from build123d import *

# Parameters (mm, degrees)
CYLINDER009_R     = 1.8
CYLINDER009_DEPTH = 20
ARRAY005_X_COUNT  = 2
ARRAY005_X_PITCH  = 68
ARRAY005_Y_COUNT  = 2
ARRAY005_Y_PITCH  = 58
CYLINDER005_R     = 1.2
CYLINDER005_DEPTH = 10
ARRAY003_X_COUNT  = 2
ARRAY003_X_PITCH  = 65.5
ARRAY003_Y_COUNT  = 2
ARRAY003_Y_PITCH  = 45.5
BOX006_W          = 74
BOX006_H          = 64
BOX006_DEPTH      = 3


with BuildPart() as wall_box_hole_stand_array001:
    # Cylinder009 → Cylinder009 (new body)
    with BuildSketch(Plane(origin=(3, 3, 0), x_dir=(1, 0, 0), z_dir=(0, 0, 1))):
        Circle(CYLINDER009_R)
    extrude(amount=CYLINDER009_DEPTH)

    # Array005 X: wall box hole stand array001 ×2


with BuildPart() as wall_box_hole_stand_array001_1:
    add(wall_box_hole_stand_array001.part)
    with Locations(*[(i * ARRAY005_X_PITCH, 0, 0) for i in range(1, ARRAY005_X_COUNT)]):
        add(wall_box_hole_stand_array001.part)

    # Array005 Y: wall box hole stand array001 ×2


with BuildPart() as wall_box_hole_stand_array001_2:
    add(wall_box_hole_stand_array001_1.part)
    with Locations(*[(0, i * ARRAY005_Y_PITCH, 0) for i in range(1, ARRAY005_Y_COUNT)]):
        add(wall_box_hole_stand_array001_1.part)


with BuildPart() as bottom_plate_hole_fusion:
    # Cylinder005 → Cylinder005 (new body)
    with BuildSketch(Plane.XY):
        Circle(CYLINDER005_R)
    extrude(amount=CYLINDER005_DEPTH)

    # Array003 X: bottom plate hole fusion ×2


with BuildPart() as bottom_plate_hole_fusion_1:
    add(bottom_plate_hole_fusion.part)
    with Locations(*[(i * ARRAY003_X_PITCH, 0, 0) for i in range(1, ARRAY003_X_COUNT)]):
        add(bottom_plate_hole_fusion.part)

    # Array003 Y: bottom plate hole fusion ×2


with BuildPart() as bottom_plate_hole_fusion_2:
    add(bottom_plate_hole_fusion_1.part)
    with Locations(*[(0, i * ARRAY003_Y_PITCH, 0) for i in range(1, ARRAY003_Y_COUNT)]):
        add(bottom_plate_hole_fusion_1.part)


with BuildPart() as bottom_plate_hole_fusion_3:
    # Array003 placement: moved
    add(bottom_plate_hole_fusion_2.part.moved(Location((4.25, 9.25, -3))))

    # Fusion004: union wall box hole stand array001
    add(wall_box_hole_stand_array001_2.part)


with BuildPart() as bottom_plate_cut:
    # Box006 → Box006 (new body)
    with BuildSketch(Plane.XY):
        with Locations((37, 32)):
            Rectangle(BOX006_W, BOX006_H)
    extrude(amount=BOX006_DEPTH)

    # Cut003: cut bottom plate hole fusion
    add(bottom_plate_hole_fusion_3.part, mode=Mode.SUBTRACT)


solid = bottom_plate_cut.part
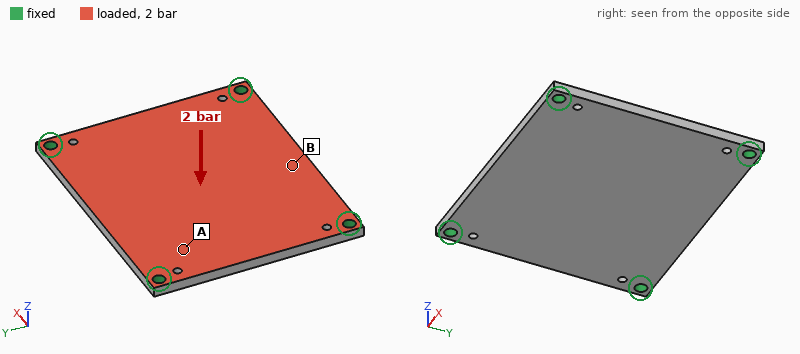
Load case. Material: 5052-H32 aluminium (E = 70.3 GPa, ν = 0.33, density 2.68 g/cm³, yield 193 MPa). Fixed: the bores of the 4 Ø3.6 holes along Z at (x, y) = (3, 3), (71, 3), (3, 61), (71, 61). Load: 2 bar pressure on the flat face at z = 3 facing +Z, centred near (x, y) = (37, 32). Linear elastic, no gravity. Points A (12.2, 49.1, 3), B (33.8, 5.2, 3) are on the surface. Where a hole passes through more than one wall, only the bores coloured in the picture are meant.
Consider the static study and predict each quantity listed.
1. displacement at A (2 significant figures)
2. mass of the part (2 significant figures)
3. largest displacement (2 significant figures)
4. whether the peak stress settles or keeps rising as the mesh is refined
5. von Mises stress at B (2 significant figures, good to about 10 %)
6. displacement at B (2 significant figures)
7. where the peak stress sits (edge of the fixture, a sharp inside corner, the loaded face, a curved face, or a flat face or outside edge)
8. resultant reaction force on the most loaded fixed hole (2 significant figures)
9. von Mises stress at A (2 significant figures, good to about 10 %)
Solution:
0.064 mm
38 g
0.16 mm
keeps rising
36 MPa
0.12 mm
edge of the fixture
230 N
12 MPa
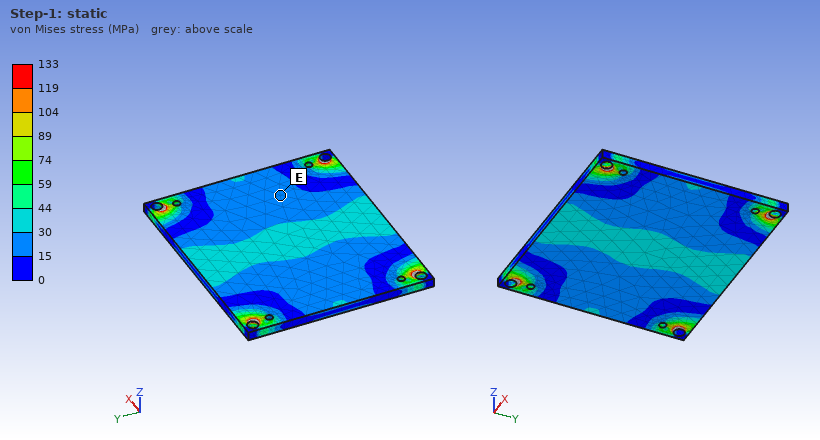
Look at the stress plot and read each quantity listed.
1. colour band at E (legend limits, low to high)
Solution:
15 to 30 MPa
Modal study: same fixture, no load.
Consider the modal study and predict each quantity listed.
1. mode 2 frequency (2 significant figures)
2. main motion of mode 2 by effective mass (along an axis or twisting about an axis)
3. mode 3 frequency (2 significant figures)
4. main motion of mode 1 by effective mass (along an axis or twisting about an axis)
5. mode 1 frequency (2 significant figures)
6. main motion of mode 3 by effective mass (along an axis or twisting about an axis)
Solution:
4000 Hz
twisting about X
4700 Hz
along Z
2400 Hz
twisting about Y
